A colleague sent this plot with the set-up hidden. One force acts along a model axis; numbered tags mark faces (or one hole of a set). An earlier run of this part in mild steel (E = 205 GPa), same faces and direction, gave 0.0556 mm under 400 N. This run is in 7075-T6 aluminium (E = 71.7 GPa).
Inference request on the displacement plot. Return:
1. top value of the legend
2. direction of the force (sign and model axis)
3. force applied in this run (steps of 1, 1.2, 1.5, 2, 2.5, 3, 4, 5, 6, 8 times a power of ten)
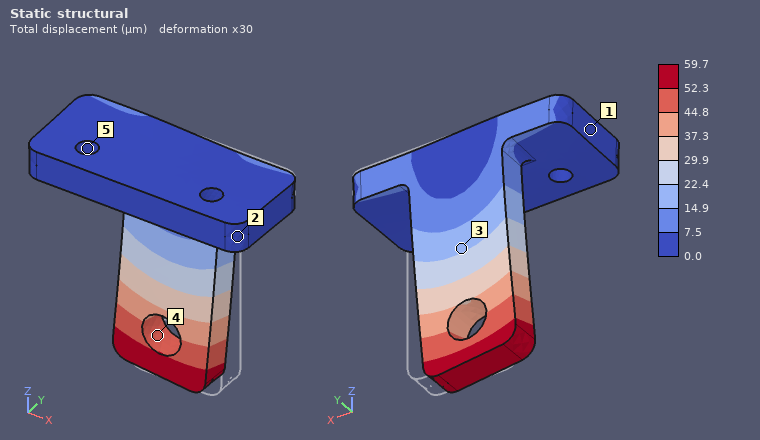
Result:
59.7 µm
-X
150 N
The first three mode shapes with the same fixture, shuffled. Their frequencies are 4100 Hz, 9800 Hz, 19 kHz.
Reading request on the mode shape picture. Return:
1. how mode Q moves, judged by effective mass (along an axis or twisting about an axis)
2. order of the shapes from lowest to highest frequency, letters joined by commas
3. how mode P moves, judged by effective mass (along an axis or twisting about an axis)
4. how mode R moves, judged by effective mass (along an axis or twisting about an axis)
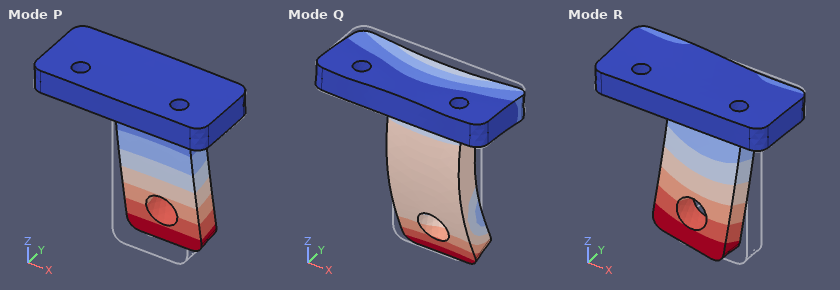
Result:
along Z
P, R, Q
along Y
along X
